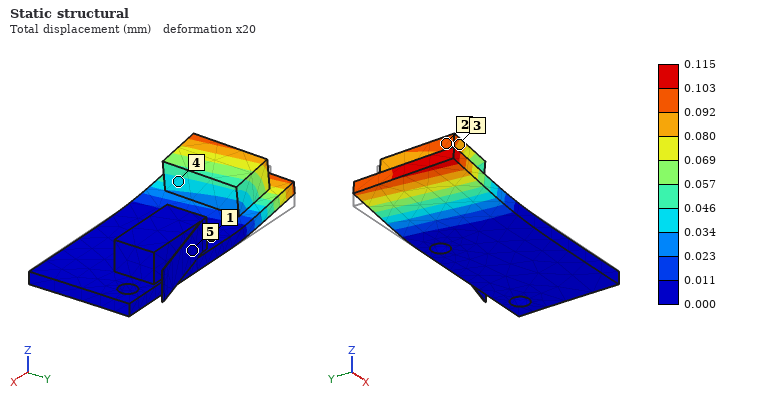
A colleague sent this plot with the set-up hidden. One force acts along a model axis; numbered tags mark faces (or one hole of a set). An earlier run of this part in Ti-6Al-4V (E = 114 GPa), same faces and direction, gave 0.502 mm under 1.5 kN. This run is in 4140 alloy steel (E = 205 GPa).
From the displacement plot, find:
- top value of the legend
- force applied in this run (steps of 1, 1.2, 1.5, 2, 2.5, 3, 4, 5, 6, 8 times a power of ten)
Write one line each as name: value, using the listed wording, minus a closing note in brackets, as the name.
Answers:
top value of the legend: 0.115 mm
force applied in this run: 600 N
